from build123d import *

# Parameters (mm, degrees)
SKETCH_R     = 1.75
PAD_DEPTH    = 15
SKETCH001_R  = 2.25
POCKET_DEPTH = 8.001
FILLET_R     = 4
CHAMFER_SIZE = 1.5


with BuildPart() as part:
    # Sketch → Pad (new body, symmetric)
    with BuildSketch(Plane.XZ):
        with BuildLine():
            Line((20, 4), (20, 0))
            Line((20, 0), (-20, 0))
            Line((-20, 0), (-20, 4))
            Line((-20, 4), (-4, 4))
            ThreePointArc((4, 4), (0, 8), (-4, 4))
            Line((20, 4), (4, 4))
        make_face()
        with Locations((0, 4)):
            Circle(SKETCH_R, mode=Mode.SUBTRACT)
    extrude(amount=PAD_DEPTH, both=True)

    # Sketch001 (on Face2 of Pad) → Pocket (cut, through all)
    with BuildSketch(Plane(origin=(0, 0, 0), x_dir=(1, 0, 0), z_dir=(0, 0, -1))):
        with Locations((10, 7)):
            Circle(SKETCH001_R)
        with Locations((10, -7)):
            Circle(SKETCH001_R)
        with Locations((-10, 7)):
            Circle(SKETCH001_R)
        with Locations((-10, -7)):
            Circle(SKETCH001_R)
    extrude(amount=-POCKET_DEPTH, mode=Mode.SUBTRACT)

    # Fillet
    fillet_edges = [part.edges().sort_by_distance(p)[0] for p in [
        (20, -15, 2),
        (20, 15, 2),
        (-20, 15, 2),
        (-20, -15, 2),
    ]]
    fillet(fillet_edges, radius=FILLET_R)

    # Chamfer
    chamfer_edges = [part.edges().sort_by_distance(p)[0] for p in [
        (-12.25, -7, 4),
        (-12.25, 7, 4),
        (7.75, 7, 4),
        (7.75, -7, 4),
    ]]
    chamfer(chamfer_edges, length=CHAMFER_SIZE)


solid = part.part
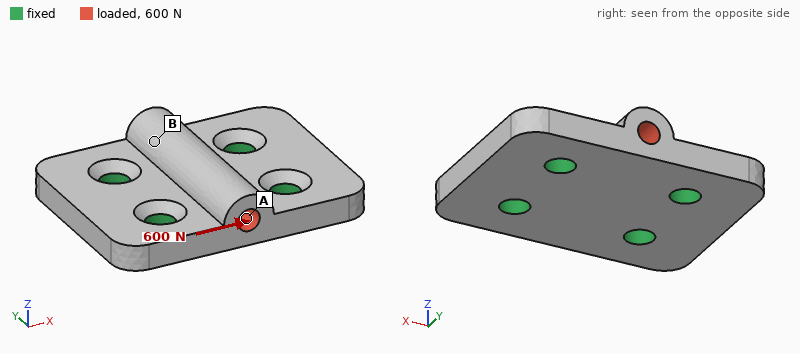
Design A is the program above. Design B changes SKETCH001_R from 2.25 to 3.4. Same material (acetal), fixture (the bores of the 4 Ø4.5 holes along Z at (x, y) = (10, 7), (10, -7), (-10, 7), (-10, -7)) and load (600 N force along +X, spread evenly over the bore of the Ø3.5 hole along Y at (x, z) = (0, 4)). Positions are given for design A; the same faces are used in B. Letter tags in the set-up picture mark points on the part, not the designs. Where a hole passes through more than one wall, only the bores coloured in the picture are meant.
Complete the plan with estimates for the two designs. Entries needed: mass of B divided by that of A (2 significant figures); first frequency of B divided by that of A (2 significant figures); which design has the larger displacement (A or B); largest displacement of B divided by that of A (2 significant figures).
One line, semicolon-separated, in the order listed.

0.93; 1.3; A; 0.86
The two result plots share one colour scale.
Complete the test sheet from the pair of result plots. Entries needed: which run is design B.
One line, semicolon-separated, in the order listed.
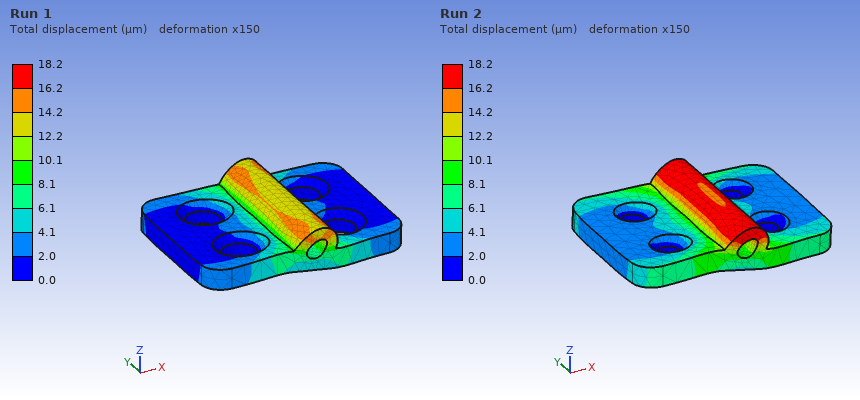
Run 1
